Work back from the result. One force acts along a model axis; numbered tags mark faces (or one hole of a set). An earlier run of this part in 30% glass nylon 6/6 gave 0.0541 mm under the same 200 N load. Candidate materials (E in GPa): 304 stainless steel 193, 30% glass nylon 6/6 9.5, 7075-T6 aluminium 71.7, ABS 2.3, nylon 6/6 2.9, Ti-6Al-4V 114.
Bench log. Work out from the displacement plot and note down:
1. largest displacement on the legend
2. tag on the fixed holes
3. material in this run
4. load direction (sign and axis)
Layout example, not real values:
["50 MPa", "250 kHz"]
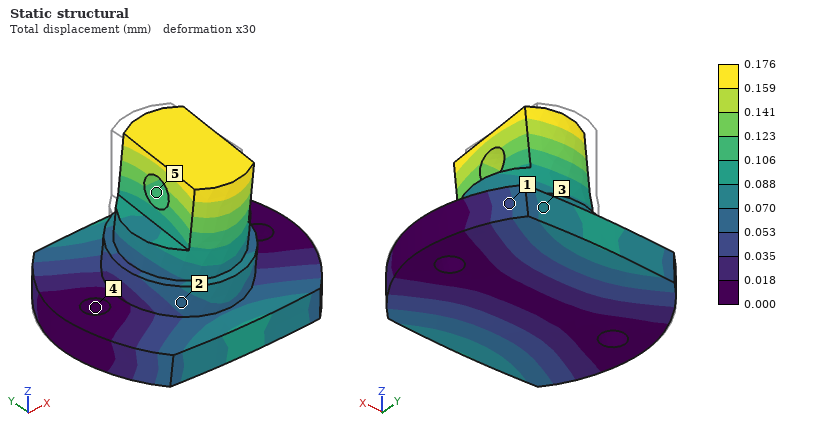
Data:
["0.176 mm", "4", "nylon 6/6", "-Y"]
